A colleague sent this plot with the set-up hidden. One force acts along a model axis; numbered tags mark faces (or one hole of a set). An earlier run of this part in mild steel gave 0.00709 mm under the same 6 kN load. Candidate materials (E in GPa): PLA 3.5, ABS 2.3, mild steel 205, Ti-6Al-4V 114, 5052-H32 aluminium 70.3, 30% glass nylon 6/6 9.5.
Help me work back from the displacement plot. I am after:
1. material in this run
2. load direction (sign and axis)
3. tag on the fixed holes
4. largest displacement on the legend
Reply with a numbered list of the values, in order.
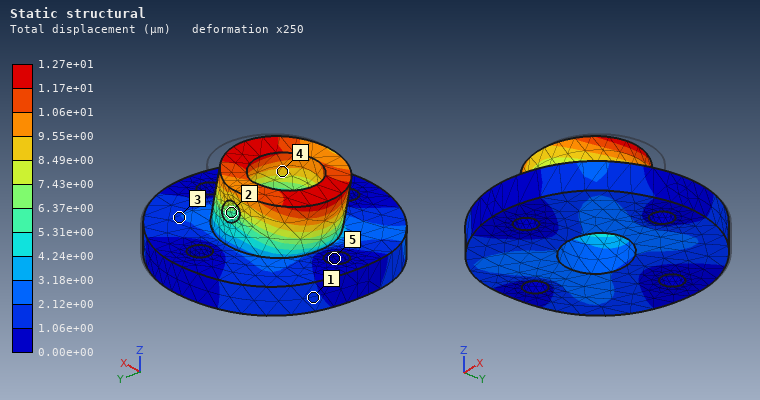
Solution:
1. Ti-6Al-4V
2. -X
3. 5
4. 1.27e+01 µm
